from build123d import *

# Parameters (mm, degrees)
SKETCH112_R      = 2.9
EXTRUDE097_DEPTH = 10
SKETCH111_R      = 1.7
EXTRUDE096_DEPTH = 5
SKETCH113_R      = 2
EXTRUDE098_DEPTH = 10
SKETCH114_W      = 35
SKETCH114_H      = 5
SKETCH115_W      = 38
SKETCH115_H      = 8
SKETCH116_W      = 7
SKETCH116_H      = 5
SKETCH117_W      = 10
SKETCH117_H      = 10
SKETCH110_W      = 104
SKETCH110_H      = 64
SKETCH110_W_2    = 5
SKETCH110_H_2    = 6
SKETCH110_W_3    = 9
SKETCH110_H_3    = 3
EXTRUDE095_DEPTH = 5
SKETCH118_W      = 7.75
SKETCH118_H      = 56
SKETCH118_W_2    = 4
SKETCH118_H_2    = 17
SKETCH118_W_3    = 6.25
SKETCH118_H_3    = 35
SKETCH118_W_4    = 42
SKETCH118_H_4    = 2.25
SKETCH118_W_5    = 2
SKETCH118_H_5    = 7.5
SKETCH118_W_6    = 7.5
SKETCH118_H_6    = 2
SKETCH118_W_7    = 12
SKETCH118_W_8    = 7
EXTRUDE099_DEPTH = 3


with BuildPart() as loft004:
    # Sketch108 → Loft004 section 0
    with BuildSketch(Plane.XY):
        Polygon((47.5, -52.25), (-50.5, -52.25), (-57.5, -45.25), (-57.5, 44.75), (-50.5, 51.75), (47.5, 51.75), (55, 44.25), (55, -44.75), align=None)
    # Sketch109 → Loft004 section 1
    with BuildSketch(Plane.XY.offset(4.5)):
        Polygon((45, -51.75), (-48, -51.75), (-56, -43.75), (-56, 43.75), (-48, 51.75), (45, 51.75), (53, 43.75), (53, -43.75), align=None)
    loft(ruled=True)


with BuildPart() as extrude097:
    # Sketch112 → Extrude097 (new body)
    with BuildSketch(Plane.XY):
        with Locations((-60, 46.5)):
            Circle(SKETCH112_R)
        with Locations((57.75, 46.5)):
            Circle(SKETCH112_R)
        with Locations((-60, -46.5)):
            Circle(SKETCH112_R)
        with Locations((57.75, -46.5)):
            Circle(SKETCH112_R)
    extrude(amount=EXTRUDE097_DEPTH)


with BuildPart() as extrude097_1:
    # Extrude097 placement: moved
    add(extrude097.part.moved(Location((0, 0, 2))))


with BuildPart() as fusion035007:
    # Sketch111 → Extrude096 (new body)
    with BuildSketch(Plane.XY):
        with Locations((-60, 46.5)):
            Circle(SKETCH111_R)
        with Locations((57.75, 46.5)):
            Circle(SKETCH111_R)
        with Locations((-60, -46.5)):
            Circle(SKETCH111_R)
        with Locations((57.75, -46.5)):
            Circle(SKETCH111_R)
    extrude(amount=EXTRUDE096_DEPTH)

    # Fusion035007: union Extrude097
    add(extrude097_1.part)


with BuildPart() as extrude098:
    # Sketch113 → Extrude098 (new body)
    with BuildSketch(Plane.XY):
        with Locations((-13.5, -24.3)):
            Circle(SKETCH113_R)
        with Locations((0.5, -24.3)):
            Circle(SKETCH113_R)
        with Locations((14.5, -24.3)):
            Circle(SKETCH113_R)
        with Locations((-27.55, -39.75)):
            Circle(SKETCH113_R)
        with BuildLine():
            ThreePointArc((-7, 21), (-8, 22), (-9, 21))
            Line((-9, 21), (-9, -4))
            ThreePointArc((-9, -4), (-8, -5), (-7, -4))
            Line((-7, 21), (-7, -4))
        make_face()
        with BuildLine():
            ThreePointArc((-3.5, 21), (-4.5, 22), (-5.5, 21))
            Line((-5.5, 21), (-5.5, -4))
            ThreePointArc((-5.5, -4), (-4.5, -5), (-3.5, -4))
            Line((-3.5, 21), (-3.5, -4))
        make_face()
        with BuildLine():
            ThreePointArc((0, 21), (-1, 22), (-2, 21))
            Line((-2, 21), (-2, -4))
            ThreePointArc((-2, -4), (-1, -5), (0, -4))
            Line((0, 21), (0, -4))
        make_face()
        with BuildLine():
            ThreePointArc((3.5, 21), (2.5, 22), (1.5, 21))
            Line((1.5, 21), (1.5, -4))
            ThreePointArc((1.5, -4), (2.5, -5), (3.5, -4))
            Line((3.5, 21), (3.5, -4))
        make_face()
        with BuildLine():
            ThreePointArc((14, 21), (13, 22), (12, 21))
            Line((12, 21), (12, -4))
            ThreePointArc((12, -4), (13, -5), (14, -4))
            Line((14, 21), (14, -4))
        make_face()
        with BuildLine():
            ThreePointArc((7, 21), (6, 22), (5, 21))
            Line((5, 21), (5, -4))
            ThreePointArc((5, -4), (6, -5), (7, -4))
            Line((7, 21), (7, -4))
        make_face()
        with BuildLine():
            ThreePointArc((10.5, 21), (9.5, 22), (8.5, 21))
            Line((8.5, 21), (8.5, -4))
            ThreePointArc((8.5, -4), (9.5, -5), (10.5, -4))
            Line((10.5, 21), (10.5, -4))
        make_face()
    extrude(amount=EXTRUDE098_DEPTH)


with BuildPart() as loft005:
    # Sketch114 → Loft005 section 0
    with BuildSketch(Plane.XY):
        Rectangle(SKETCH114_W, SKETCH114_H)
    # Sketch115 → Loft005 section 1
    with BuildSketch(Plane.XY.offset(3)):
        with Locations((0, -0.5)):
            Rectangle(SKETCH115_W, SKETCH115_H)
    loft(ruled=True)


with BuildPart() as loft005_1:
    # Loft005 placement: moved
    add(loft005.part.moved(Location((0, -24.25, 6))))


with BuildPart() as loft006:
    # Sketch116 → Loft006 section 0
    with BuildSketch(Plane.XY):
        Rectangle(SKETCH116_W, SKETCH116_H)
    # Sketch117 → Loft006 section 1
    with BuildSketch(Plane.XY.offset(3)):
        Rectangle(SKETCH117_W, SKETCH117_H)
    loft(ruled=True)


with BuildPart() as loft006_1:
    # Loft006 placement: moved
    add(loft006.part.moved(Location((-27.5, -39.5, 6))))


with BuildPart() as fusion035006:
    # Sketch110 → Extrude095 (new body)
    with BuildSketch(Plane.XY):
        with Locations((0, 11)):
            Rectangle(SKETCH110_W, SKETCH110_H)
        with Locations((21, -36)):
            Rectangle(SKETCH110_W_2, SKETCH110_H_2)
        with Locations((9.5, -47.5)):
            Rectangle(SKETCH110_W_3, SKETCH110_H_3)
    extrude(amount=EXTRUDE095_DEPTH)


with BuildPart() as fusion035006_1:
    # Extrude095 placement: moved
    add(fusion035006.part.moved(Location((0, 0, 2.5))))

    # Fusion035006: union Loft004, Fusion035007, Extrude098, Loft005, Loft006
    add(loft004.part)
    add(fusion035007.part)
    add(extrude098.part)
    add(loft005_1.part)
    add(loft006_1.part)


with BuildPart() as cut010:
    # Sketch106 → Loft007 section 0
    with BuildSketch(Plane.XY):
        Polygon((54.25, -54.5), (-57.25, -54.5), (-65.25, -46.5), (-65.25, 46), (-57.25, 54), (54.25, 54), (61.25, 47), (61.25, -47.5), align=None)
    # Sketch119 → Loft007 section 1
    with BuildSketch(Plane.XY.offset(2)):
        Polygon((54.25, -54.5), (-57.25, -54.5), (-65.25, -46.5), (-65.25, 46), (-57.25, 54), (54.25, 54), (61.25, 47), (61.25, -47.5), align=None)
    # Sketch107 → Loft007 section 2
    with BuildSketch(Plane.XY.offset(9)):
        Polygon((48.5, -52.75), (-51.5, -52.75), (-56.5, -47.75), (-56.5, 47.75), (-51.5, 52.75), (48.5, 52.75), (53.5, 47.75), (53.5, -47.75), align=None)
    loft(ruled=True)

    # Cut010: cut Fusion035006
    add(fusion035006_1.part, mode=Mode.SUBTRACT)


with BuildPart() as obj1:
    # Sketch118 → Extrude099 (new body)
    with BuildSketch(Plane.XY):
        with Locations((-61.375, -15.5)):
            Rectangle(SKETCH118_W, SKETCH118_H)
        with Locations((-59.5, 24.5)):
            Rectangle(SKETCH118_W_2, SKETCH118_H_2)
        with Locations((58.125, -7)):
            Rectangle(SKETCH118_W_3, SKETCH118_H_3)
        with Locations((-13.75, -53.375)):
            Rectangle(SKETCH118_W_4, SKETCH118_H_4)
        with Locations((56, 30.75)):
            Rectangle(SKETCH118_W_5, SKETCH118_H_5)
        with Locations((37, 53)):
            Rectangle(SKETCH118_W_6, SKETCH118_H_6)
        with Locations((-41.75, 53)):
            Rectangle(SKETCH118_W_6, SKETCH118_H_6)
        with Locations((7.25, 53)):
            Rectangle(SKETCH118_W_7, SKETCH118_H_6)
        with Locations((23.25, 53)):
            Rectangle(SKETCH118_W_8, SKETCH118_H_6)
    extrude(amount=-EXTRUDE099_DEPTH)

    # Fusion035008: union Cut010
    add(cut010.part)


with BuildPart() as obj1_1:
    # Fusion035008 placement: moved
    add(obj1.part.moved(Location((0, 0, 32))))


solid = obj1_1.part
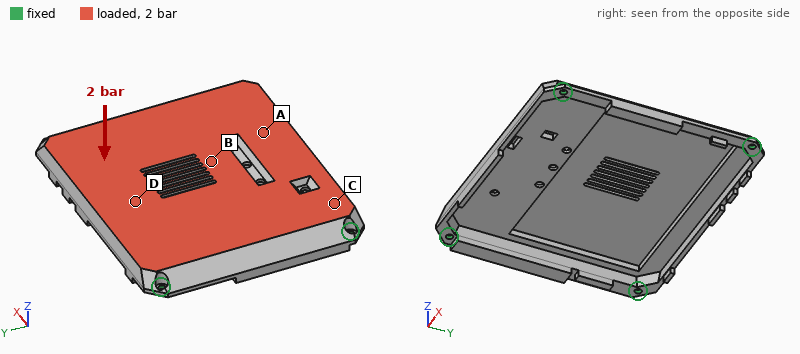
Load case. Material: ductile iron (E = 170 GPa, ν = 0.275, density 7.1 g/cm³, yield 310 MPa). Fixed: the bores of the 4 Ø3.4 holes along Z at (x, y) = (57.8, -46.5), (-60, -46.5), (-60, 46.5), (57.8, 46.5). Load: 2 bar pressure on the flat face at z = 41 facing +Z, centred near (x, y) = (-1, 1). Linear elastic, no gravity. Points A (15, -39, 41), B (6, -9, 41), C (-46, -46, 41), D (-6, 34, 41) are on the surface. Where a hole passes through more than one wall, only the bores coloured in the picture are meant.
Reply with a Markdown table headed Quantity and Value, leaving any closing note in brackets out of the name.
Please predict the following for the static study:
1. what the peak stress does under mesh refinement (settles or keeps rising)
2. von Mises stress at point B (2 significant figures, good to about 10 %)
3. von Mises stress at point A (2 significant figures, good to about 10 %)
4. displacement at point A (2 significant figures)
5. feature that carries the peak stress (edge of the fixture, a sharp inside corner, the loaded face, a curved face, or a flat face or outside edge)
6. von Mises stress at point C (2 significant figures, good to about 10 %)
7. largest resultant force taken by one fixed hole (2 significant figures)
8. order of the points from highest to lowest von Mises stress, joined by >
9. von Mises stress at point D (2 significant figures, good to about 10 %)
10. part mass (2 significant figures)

| Quantity | Value |
|---|---|
| what the peak stress does under mesh refinement | keeps rising |
| von Mises stress at point B | 79 MPa |
| von Mises stress at point A | 47 MPa |
| displacement at point A | 0.093 mm |
| feature that carries the peak stress | edge of the fixture |
| von Mises stress at point C | 27 MPa |
| largest resultant force taken by one fixed hole | 1.7 kN |
| order of the points from highest to lowest von Mises stress, joined by > | B > D > A > C |
| von Mises stress at point D | 60 MPa |
| part mass | 320 g |
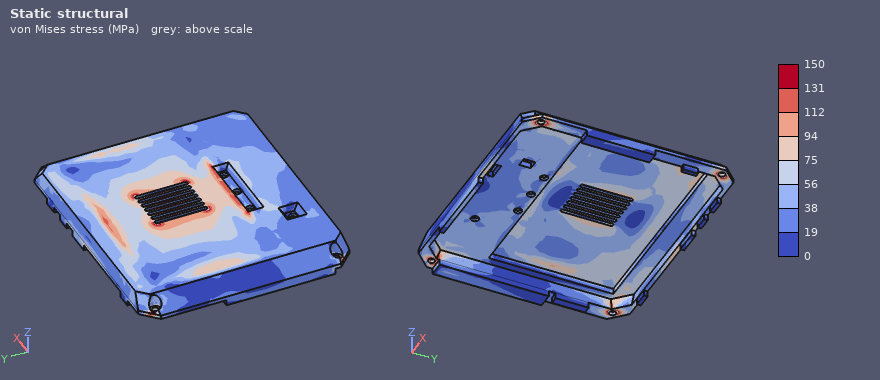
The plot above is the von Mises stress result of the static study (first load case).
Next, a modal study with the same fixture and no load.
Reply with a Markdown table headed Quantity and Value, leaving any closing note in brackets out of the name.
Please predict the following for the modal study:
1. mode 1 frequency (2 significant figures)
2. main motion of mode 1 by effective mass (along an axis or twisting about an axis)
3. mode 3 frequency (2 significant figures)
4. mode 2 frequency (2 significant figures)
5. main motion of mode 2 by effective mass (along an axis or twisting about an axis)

| Quantity | Value |
|---|---|
| mode 1 frequency | 1400 Hz |
| main motion of mode 1 by effective mass | along Z |
| mode 3 frequency | 2400 Hz |
| mode 2 frequency | 1900 Hz |
| main motion of mode 2 by effective mass | twisting about X |
